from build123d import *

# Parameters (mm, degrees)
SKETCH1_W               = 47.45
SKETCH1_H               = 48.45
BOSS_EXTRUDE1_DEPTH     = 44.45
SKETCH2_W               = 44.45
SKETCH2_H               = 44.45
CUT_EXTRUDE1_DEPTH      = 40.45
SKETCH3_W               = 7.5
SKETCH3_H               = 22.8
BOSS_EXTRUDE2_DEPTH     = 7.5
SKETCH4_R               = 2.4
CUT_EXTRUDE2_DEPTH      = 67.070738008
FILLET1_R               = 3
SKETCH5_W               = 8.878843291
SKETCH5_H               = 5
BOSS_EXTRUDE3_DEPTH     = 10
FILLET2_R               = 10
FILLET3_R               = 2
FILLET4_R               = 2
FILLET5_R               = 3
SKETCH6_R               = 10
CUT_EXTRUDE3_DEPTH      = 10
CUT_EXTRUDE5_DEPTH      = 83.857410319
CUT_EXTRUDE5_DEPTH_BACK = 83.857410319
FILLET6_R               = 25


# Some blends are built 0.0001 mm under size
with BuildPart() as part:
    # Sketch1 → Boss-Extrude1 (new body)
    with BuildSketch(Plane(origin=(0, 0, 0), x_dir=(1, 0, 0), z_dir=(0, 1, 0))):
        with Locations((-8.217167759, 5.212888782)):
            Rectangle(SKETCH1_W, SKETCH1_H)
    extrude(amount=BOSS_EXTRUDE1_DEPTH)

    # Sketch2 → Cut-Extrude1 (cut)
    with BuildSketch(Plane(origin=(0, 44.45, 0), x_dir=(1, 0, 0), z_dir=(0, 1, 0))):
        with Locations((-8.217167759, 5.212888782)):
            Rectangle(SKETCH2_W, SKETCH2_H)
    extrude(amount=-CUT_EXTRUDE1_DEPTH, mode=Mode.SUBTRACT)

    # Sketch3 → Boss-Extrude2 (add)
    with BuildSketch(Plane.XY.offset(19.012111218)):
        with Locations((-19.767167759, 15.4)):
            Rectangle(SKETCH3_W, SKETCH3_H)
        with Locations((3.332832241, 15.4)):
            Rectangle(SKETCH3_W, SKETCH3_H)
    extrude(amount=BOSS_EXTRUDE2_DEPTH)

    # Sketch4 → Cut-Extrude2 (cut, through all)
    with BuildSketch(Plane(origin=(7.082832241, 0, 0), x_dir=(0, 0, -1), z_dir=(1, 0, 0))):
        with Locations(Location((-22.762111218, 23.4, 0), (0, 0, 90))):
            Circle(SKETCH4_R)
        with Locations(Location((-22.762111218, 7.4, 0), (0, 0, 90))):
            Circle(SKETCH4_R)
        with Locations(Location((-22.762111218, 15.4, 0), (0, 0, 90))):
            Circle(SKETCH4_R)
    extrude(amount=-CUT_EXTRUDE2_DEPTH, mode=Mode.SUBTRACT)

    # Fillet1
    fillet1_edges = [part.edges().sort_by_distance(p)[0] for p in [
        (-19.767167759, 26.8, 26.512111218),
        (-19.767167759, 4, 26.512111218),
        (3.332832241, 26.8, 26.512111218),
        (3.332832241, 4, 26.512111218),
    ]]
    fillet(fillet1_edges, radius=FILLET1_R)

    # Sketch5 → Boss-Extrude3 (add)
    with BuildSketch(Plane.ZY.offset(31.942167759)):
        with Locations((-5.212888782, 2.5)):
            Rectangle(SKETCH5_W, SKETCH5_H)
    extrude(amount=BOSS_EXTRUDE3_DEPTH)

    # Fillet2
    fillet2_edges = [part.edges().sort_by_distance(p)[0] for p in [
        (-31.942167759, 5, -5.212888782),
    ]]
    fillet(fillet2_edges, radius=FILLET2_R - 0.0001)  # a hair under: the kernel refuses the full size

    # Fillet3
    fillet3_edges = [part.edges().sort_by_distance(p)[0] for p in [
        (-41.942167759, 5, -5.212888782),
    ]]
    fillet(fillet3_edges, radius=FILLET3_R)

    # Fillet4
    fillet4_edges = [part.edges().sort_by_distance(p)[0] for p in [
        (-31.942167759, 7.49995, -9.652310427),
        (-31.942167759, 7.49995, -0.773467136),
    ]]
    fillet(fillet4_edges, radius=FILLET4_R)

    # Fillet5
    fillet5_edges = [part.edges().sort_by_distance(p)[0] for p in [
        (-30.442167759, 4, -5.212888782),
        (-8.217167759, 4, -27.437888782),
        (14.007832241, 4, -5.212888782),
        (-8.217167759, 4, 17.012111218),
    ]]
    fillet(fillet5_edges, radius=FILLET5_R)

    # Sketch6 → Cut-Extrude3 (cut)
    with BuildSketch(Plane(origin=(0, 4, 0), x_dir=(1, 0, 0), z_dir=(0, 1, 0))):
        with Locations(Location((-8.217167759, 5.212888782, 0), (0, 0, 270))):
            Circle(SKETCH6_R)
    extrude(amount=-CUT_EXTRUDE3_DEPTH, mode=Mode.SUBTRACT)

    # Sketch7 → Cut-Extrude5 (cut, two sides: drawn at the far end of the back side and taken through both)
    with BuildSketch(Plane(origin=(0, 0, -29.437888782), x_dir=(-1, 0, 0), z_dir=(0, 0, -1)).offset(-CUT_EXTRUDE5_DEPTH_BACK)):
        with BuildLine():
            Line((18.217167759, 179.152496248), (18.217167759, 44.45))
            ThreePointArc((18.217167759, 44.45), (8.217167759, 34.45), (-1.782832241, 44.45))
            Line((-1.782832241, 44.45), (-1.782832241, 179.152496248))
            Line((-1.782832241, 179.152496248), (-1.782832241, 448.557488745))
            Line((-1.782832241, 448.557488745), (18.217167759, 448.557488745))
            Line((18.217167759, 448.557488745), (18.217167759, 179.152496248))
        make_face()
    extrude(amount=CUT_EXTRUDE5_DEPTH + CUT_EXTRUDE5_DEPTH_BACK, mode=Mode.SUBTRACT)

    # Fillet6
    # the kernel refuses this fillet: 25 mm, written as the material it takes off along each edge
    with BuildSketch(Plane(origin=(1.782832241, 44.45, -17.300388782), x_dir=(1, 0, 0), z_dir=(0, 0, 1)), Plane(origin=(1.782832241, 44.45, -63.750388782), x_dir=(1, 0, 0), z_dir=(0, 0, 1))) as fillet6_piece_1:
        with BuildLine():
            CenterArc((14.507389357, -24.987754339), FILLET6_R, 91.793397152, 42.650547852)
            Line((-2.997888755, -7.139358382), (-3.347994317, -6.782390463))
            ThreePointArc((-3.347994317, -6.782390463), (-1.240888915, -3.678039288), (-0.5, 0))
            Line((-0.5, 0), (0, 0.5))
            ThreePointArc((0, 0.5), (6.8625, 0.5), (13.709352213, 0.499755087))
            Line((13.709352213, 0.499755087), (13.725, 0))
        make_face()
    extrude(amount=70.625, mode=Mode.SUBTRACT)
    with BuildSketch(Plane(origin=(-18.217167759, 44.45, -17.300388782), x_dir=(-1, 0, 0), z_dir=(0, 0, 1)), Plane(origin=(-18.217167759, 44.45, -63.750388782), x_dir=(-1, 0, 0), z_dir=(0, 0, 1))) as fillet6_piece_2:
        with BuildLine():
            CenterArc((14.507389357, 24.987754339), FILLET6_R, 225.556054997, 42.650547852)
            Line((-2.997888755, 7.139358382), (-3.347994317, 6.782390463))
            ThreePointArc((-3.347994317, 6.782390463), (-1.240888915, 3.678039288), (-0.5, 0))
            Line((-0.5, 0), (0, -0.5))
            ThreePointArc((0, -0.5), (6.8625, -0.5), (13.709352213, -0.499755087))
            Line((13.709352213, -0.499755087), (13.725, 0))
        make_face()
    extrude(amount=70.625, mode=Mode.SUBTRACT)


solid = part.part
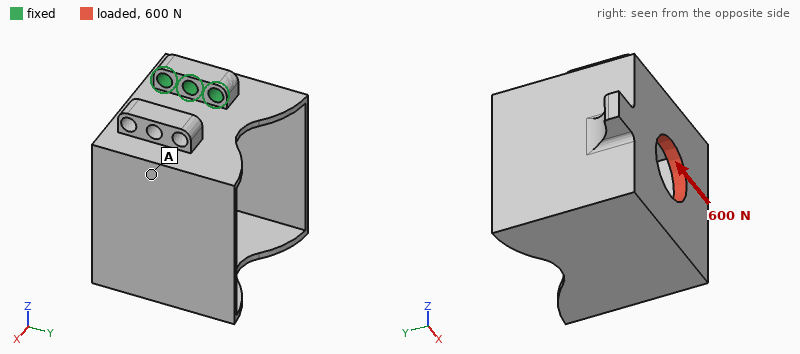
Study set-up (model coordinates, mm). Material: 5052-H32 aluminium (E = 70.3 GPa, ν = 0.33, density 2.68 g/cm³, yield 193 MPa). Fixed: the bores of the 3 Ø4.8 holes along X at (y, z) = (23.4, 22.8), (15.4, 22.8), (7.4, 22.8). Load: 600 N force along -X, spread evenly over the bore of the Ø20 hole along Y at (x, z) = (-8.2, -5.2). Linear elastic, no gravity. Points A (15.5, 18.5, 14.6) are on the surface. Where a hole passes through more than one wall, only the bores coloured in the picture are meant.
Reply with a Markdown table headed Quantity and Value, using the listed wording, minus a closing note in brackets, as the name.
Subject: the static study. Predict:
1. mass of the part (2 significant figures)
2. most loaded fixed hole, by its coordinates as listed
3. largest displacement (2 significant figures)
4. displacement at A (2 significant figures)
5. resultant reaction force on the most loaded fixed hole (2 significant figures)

| Quantity | Value |
|---|---|
| mass of the part | 61 g |
| most loaded fixed hole, by its coordinates as listed | (7.4, 22.8) |
| largest displacement | 0.46 mm |
| displacement at A | 0.24 mm |
| resultant reaction force on the most loaded fixed hole | 440 N |
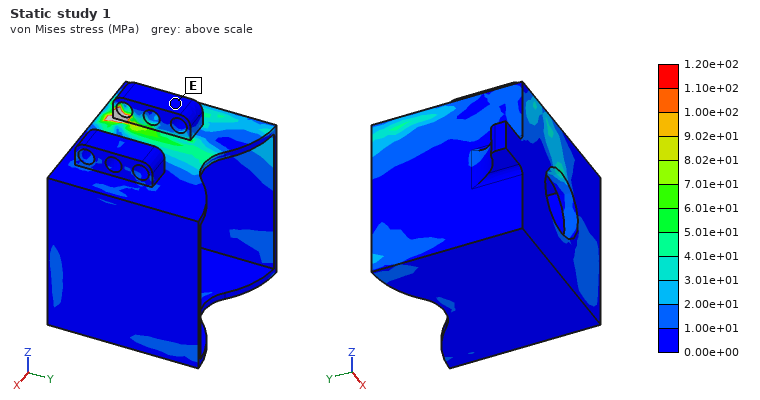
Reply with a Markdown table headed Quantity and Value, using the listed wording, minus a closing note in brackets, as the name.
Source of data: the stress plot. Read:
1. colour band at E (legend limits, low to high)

| Quantity | Value |
|---|---|
| colour band at E | 0.00e+00 to 1.00e+01 MPa |
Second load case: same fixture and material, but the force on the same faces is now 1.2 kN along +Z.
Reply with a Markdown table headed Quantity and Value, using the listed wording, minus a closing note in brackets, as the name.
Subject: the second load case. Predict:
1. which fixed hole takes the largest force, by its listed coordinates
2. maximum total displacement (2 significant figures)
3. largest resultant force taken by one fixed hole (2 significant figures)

| Quantity | Value |
|---|---|
| which fixed hole takes the largest force, by its listed coordinates | (7.4, 22.8) |
| maximum total displacement | 0.45 mm |
| largest resultant force taken by one fixed hole | 1.5 kN |
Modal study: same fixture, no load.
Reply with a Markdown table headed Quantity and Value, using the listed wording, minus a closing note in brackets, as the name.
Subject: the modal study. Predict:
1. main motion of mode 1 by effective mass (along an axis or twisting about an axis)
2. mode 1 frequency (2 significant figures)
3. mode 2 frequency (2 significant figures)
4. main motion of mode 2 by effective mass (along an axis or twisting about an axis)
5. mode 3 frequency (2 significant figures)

| Quantity | Value |
|---|---|
| main motion of mode 1 by effective mass | along X |
| mode 1 frequency | 780 Hz |
| mode 2 frequency | 880 Hz |
| main motion of mode 2 by effective mass | along Y |
| mode 3 frequency | 1900 Hz |
